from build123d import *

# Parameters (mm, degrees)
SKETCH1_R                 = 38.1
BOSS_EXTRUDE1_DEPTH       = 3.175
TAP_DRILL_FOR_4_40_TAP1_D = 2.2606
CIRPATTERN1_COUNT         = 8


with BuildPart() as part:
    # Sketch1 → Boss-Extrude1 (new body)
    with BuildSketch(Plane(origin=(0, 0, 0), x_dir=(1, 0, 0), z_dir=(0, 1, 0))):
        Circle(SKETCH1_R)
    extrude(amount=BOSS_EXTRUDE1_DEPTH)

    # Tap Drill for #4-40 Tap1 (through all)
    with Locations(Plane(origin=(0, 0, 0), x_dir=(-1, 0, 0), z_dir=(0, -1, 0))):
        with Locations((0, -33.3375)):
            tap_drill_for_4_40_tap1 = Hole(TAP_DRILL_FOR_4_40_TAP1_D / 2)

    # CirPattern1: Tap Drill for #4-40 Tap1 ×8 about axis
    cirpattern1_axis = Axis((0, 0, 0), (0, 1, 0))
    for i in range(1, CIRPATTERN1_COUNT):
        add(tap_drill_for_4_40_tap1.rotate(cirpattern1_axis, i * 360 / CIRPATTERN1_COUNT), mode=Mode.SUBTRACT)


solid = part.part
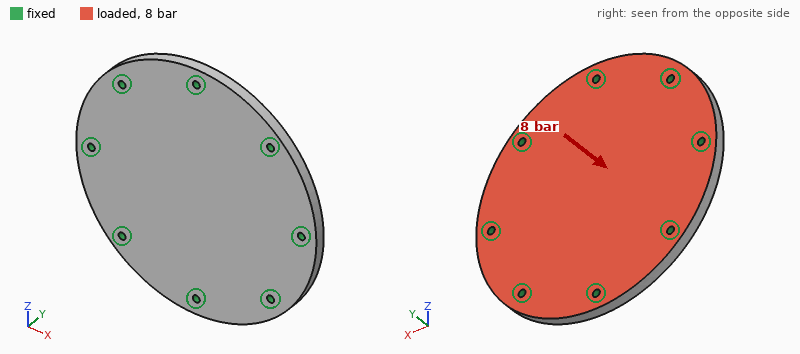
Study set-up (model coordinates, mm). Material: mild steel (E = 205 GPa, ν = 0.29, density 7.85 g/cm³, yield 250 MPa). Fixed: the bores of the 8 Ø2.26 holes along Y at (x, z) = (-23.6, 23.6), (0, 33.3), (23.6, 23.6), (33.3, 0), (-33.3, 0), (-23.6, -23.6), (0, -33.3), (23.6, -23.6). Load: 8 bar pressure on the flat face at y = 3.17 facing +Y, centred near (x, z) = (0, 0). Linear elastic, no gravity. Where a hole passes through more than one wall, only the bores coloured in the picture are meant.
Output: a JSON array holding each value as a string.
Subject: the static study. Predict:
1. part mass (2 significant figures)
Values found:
["110 g"]
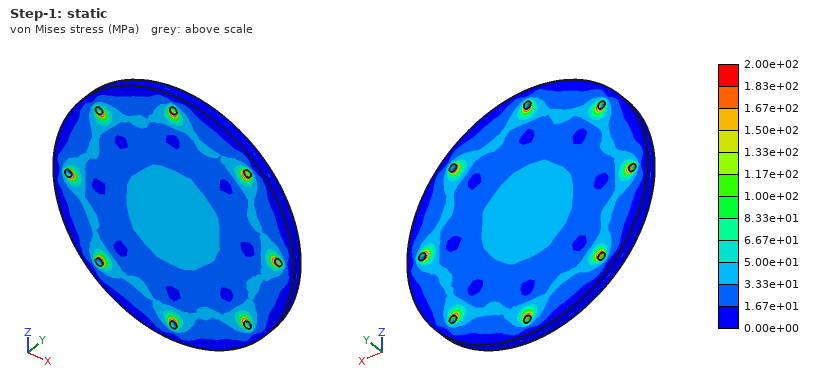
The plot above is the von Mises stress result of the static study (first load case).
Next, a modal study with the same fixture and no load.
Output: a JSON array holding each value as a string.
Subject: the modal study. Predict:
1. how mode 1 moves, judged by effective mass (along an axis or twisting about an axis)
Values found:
["along Y"]
